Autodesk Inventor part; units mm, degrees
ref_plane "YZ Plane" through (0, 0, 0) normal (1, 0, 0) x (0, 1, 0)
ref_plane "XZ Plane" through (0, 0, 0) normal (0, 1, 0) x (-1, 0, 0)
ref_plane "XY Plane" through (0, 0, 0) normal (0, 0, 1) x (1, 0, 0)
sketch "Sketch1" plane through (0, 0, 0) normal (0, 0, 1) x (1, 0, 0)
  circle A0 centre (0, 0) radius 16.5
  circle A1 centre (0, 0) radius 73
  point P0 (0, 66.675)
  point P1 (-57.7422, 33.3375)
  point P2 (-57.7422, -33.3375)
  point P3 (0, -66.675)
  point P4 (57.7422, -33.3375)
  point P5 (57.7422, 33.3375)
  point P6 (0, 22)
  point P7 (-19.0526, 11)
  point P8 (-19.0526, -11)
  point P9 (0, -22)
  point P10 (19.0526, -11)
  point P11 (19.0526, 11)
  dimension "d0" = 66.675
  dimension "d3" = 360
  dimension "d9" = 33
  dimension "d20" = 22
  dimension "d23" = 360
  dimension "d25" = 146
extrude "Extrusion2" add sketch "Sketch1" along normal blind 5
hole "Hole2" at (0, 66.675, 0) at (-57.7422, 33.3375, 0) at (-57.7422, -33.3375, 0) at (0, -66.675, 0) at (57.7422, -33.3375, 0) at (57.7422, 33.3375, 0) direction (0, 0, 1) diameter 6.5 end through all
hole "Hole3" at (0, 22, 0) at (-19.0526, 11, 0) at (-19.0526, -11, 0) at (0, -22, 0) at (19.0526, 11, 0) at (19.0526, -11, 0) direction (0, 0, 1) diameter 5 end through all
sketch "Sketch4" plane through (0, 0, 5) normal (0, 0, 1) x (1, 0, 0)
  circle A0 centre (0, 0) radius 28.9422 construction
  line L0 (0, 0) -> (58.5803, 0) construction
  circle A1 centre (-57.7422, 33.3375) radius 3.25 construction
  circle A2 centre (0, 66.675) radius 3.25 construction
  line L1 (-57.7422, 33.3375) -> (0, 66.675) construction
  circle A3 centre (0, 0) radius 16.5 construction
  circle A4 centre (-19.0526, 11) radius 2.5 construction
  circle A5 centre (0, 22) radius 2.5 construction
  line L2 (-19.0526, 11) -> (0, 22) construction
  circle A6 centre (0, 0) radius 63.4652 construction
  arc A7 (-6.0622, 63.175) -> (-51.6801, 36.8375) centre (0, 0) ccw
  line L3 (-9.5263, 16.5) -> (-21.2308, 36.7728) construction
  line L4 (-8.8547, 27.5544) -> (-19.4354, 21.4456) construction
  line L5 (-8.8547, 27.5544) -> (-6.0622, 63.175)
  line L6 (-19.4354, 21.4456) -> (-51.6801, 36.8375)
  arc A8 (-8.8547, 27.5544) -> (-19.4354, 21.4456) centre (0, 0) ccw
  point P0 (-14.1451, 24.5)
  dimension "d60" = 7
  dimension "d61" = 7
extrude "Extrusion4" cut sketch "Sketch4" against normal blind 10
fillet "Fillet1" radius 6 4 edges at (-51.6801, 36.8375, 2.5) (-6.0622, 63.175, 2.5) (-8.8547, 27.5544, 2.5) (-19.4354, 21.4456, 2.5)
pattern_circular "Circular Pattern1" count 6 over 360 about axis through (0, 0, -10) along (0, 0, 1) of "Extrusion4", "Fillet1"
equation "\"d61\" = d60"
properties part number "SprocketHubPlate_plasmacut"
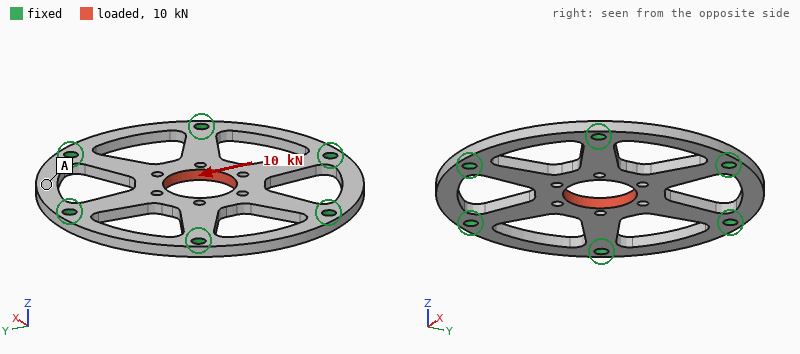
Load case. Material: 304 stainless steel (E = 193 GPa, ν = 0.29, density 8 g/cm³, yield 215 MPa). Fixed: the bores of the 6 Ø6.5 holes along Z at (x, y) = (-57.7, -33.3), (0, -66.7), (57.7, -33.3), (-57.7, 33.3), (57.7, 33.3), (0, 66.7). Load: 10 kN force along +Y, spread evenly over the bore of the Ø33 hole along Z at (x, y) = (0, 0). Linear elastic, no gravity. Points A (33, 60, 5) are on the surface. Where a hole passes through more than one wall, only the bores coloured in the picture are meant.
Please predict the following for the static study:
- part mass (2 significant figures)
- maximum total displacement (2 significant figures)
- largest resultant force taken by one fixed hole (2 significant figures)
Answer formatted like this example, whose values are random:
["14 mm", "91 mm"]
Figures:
["350 g", "10 µm", "2.9 kN"]
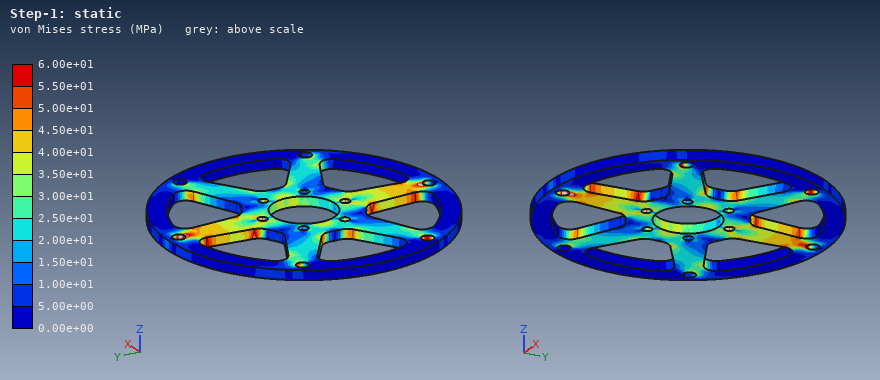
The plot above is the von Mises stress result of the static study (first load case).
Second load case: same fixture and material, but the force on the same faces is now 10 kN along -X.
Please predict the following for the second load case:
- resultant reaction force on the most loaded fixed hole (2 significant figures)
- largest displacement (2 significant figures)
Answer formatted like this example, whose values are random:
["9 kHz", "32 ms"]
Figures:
["2.6 kN", "10 µm"]
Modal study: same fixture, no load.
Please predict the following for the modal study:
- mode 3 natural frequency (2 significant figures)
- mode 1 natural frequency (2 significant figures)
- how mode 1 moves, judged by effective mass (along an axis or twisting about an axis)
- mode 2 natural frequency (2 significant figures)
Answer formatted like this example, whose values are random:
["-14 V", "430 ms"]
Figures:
["4000 Hz", "2000 Hz", "along Z", "4000 Hz"]
